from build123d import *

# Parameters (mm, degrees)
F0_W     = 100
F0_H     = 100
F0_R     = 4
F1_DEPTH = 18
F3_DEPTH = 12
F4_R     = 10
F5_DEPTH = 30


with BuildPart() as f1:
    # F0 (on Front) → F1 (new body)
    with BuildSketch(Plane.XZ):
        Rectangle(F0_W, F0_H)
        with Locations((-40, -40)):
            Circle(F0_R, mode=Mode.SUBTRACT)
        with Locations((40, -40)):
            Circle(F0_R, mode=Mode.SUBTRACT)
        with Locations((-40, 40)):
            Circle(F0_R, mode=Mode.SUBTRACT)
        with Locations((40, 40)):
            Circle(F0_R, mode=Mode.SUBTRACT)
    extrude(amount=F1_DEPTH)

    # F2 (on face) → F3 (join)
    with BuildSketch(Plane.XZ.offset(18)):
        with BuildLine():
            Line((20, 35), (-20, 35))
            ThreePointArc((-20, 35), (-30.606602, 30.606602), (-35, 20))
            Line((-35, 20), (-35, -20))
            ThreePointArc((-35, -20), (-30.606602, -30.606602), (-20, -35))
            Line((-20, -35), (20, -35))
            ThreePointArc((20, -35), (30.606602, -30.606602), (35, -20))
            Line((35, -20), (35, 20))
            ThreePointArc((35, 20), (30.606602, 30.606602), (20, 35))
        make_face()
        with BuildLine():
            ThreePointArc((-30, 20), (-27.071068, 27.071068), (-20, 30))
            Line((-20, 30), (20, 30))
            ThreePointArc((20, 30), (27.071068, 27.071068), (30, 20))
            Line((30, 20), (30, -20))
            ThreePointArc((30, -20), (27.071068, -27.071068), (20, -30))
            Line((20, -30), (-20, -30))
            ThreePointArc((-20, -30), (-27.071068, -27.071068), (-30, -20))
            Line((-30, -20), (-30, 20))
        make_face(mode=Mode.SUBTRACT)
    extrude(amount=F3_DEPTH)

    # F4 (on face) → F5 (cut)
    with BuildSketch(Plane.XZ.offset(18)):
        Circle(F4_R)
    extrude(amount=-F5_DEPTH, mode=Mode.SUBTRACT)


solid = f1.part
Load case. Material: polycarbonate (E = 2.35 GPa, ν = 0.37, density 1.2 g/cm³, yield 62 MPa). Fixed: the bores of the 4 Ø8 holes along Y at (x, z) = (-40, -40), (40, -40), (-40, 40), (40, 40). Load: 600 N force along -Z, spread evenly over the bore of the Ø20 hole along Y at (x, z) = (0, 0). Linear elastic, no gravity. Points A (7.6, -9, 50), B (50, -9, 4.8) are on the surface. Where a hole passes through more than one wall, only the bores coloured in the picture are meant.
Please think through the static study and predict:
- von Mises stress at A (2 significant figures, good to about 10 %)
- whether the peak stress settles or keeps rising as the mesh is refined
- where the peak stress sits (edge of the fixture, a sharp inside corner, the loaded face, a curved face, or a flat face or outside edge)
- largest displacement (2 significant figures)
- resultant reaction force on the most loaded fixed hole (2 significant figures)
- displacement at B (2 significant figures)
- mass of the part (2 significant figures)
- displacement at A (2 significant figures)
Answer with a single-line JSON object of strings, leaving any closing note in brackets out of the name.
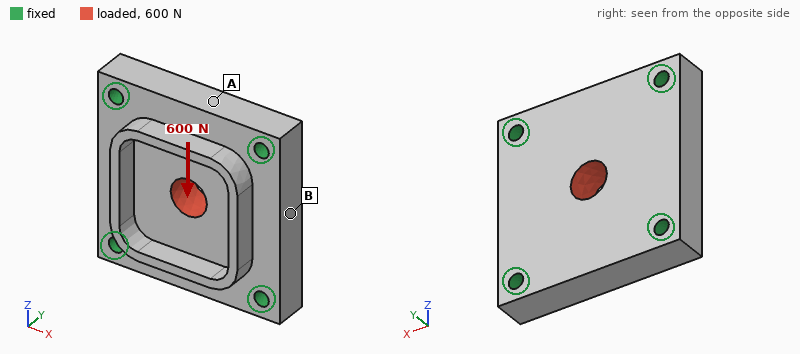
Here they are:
{"von Mises stress at A": "0.26 MPa", "whether the peak stress settles or keeps rising as the mesh is refined": "keeps rising", "where the peak stress sits": "edge of the fixture", "largest displacement": "11 µm", "resultant reaction force on the most loaded fixed hole": "170 N", "displacement at B": "1.9 µm", "mass of the part": "220 g", "displacement at A": "6.8 µm"}
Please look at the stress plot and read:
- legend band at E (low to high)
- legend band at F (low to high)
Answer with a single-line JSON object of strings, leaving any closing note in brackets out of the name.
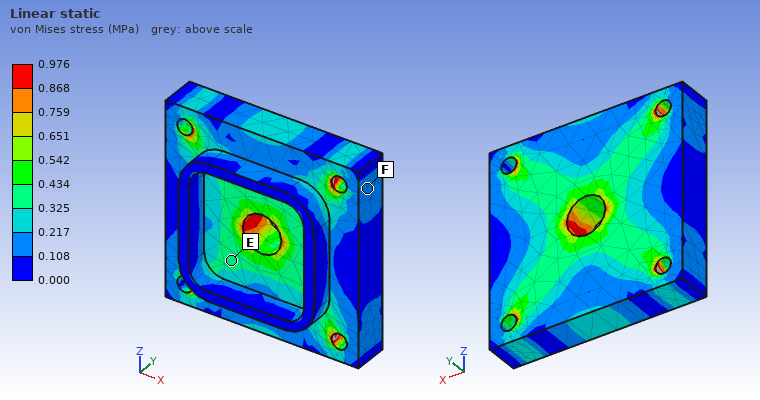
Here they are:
{"legend band at E": "0.325 to 0.434 MPa", "legend band at F": "0.108 to 0.217 MPa"}
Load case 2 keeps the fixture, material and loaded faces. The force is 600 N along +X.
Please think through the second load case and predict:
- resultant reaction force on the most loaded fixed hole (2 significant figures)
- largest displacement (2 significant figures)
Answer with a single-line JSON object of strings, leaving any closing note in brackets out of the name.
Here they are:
{"resultant reaction force on the most loaded fixed hole": "170 N", "largest displacement": "11 µm"}
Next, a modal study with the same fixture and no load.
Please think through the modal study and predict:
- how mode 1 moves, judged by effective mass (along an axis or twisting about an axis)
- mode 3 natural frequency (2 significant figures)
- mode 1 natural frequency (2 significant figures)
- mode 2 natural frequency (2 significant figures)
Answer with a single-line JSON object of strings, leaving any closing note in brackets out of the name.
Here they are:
{"how mode 1 moves, judged by effective mass": "along Y", "mode 3 natural frequency": "3400 Hz", "mode 1 natural frequency": "2300 Hz", "mode 2 natural frequency": "3400 Hz"}
